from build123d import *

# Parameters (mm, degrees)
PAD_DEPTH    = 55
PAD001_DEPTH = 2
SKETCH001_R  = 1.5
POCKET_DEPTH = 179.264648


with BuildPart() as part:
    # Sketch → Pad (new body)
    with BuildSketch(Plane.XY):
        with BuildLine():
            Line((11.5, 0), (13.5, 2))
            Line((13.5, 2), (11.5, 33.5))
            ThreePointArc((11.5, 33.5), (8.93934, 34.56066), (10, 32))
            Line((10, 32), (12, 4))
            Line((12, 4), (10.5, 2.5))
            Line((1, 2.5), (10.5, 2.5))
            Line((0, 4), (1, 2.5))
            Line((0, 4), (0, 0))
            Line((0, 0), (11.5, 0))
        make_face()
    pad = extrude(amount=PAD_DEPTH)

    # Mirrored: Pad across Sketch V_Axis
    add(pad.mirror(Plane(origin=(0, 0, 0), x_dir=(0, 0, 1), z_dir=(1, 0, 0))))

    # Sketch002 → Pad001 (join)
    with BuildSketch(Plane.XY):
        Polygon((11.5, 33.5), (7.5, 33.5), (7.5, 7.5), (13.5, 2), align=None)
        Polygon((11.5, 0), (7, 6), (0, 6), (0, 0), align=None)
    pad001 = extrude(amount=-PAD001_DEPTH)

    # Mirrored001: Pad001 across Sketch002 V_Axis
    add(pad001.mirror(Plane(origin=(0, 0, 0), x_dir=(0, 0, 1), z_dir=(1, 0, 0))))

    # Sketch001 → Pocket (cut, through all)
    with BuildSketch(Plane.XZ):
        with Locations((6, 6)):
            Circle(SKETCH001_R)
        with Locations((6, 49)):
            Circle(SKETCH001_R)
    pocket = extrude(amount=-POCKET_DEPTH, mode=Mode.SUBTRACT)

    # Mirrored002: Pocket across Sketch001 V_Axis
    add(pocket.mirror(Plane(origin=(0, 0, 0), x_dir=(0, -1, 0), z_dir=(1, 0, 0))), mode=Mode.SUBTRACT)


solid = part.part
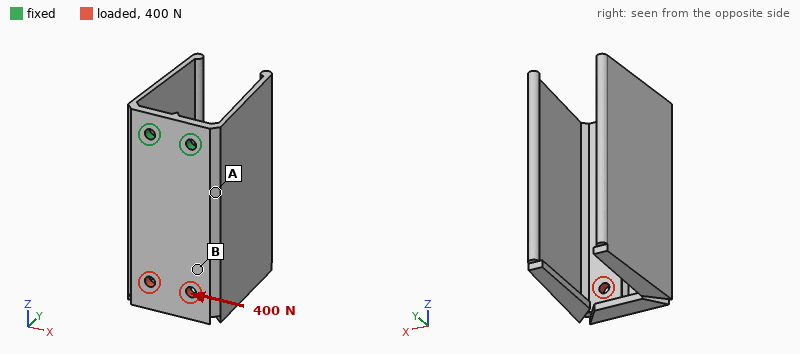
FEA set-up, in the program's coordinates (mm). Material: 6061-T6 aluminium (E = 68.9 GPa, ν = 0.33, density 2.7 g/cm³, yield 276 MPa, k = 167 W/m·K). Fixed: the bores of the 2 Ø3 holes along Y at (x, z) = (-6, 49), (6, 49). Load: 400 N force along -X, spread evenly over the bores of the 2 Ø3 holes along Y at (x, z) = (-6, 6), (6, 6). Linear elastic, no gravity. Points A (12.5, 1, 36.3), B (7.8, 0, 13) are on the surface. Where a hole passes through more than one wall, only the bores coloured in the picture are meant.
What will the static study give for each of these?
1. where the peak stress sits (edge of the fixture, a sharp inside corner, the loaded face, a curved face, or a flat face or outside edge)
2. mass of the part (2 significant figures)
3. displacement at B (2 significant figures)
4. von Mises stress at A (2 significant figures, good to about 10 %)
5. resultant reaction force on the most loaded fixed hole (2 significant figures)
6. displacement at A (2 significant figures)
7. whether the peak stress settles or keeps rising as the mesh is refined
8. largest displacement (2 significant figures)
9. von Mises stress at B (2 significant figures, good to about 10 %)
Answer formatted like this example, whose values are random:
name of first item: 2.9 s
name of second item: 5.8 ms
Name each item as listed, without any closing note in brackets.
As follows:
where the peak stress sits: edge of the fixture
mass of the part: 27 g
displacement at B: 49 µm
von Mises stress at A: 23 MPa
resultant reaction force on the most loaded fixed hole: 1.2 kN
displacement at A: 19 µm
whether the peak stress settles or keeps rising as the mesh is refined: keeps rising
largest displacement: 74 µm
von Mises stress at B: 9.6 MPa
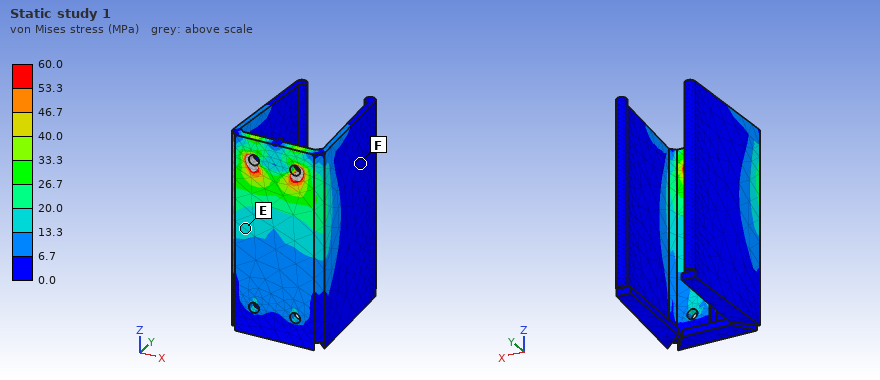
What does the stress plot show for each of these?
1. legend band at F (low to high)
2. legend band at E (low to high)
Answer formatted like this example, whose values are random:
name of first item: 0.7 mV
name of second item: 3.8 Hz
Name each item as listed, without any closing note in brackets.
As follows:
legend band at F: 0.0 to 6.7 MPa
legend band at E: 13.3 to 20.0 MPa
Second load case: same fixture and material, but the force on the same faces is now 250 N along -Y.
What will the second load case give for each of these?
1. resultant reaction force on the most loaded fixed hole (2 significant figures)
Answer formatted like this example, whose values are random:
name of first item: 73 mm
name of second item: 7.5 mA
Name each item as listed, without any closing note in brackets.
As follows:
resultant reaction force on the most loaded fixed hole: 130 N
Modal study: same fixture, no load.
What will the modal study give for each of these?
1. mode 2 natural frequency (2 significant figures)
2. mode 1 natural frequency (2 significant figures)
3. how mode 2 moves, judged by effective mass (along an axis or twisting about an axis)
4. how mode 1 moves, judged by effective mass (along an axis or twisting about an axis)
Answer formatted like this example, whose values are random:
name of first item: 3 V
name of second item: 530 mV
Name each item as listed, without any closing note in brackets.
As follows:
mode 2 natural frequency: 840 Hz
mode 1 natural frequency: 730 Hz
how mode 2 moves, judged by effective mass: along Y
how mode 1 moves, judged by effective mass: along X
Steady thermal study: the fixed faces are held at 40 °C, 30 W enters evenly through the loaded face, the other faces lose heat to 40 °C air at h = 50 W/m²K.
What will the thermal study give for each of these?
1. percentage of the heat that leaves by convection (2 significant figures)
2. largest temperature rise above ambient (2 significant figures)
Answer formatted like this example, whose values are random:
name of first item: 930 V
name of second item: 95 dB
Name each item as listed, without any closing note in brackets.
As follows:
percentage of the heat that leaves by convection: 45 %
largest temperature rise above ambient: 58 K
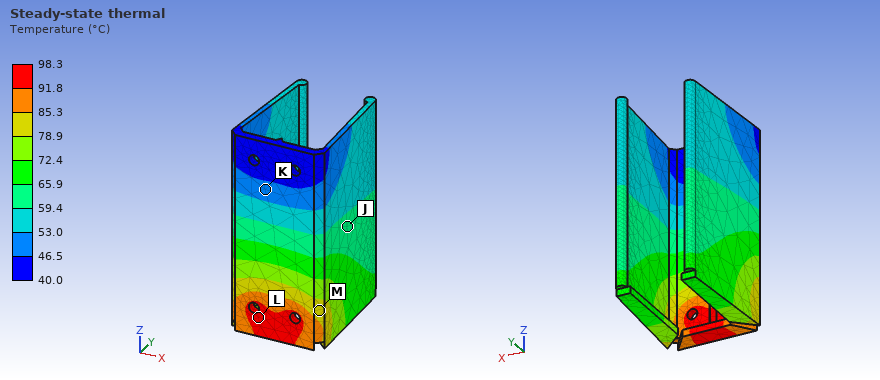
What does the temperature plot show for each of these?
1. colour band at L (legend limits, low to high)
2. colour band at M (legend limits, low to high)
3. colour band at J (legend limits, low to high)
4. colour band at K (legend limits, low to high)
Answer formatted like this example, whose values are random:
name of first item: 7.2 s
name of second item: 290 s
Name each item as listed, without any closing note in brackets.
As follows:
colour band at L: 91.8 to 98.3 °C
colour band at M: 78.9 to 85.3 °C
colour band at J: 59.4 to 65.9 °C
colour band at K: 46.5 to 53.0 °C
